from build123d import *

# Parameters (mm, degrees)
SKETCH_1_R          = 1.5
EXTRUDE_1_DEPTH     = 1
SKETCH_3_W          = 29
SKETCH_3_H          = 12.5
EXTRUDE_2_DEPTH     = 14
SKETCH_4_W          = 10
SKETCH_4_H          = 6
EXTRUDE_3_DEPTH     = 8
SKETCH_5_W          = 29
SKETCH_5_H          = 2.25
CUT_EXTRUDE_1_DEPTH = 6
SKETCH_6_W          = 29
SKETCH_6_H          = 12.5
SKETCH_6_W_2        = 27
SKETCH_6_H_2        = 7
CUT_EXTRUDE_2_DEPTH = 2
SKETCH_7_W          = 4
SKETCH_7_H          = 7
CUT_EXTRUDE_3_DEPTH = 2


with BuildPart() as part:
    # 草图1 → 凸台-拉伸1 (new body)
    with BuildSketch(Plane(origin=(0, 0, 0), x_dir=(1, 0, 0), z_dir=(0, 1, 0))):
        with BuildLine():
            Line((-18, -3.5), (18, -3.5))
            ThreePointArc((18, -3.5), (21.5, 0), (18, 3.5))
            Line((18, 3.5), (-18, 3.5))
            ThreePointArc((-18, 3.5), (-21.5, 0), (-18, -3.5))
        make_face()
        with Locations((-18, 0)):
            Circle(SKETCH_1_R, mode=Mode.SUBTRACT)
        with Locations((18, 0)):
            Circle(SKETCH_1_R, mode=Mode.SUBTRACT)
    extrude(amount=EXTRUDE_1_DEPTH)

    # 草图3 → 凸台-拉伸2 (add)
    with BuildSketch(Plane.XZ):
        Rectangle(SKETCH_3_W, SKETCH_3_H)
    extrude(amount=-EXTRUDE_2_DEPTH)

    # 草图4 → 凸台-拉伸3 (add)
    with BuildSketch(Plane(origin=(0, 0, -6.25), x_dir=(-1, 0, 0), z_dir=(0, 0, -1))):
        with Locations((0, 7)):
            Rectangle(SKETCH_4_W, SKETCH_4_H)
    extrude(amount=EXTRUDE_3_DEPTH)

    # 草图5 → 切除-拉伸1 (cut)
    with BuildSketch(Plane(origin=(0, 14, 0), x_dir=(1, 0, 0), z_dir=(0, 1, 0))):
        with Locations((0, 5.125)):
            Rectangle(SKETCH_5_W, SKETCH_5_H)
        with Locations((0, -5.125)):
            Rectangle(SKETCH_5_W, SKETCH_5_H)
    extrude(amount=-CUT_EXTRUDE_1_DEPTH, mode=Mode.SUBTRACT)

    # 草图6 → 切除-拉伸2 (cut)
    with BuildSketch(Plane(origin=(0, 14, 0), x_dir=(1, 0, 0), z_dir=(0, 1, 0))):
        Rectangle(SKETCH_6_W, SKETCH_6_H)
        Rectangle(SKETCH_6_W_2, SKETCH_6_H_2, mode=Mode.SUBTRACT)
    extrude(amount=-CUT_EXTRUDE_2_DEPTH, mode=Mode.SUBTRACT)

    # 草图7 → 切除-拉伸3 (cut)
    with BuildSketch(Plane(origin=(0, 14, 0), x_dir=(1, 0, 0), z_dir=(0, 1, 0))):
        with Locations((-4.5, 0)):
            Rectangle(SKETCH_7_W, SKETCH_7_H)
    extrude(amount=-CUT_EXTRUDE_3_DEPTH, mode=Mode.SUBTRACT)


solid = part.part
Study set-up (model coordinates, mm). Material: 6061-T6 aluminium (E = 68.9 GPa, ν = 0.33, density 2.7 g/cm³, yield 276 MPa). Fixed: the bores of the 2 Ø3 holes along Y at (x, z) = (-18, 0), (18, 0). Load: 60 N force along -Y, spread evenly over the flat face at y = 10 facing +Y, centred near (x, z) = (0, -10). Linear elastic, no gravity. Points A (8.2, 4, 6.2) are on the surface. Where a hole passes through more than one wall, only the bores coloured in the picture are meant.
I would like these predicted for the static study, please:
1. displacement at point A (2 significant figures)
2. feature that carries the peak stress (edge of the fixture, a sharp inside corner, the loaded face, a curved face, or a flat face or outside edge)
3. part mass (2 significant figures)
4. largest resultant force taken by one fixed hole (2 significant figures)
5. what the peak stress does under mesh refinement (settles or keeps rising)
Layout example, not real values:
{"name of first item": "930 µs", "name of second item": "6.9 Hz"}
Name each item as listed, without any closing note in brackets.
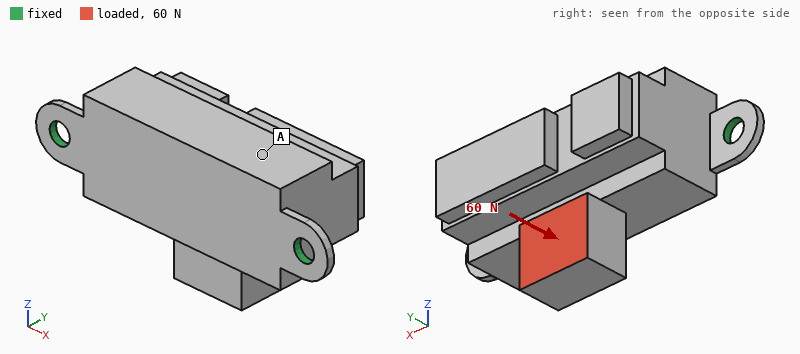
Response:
{"displacement at point A": "0.046 mm", "feature that carries the peak stress": "edge of the fixture", "part mass": "13 g", "largest resultant force taken by one fixed hole": "38 N", "what the peak stress does under mesh refinement": "keeps rising"}
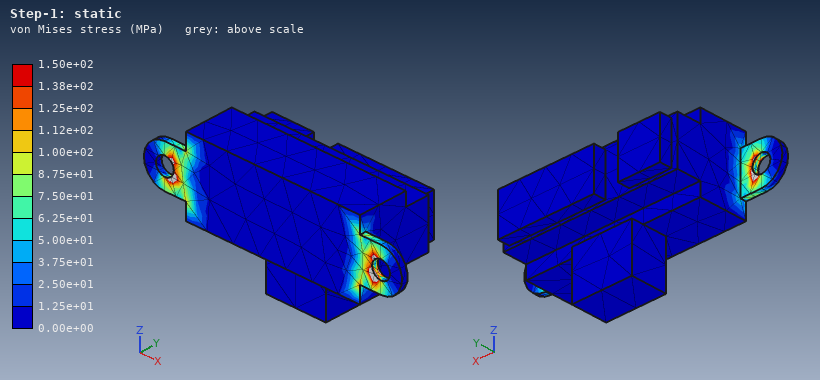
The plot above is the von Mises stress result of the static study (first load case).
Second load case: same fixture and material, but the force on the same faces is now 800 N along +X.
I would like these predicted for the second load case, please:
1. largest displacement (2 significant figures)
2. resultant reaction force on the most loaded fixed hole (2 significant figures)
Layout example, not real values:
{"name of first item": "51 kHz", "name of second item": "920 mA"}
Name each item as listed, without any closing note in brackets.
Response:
{"largest displacement": "36 µm", "resultant reaction force on the most loaded fixed hole": "530 N"}
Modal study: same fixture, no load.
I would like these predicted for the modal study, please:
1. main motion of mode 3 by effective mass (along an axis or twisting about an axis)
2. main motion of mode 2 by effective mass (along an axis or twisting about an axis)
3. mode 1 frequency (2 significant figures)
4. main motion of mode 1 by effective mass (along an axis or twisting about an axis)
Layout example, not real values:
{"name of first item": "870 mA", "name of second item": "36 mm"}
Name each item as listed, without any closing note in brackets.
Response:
{"main motion of mode 3 by effective mass": "along X", "main motion of mode 2 by effective mass": "along Y", "mode 1 frequency": "1700 Hz", "main motion of mode 1 by effective mass": "along Z"}
